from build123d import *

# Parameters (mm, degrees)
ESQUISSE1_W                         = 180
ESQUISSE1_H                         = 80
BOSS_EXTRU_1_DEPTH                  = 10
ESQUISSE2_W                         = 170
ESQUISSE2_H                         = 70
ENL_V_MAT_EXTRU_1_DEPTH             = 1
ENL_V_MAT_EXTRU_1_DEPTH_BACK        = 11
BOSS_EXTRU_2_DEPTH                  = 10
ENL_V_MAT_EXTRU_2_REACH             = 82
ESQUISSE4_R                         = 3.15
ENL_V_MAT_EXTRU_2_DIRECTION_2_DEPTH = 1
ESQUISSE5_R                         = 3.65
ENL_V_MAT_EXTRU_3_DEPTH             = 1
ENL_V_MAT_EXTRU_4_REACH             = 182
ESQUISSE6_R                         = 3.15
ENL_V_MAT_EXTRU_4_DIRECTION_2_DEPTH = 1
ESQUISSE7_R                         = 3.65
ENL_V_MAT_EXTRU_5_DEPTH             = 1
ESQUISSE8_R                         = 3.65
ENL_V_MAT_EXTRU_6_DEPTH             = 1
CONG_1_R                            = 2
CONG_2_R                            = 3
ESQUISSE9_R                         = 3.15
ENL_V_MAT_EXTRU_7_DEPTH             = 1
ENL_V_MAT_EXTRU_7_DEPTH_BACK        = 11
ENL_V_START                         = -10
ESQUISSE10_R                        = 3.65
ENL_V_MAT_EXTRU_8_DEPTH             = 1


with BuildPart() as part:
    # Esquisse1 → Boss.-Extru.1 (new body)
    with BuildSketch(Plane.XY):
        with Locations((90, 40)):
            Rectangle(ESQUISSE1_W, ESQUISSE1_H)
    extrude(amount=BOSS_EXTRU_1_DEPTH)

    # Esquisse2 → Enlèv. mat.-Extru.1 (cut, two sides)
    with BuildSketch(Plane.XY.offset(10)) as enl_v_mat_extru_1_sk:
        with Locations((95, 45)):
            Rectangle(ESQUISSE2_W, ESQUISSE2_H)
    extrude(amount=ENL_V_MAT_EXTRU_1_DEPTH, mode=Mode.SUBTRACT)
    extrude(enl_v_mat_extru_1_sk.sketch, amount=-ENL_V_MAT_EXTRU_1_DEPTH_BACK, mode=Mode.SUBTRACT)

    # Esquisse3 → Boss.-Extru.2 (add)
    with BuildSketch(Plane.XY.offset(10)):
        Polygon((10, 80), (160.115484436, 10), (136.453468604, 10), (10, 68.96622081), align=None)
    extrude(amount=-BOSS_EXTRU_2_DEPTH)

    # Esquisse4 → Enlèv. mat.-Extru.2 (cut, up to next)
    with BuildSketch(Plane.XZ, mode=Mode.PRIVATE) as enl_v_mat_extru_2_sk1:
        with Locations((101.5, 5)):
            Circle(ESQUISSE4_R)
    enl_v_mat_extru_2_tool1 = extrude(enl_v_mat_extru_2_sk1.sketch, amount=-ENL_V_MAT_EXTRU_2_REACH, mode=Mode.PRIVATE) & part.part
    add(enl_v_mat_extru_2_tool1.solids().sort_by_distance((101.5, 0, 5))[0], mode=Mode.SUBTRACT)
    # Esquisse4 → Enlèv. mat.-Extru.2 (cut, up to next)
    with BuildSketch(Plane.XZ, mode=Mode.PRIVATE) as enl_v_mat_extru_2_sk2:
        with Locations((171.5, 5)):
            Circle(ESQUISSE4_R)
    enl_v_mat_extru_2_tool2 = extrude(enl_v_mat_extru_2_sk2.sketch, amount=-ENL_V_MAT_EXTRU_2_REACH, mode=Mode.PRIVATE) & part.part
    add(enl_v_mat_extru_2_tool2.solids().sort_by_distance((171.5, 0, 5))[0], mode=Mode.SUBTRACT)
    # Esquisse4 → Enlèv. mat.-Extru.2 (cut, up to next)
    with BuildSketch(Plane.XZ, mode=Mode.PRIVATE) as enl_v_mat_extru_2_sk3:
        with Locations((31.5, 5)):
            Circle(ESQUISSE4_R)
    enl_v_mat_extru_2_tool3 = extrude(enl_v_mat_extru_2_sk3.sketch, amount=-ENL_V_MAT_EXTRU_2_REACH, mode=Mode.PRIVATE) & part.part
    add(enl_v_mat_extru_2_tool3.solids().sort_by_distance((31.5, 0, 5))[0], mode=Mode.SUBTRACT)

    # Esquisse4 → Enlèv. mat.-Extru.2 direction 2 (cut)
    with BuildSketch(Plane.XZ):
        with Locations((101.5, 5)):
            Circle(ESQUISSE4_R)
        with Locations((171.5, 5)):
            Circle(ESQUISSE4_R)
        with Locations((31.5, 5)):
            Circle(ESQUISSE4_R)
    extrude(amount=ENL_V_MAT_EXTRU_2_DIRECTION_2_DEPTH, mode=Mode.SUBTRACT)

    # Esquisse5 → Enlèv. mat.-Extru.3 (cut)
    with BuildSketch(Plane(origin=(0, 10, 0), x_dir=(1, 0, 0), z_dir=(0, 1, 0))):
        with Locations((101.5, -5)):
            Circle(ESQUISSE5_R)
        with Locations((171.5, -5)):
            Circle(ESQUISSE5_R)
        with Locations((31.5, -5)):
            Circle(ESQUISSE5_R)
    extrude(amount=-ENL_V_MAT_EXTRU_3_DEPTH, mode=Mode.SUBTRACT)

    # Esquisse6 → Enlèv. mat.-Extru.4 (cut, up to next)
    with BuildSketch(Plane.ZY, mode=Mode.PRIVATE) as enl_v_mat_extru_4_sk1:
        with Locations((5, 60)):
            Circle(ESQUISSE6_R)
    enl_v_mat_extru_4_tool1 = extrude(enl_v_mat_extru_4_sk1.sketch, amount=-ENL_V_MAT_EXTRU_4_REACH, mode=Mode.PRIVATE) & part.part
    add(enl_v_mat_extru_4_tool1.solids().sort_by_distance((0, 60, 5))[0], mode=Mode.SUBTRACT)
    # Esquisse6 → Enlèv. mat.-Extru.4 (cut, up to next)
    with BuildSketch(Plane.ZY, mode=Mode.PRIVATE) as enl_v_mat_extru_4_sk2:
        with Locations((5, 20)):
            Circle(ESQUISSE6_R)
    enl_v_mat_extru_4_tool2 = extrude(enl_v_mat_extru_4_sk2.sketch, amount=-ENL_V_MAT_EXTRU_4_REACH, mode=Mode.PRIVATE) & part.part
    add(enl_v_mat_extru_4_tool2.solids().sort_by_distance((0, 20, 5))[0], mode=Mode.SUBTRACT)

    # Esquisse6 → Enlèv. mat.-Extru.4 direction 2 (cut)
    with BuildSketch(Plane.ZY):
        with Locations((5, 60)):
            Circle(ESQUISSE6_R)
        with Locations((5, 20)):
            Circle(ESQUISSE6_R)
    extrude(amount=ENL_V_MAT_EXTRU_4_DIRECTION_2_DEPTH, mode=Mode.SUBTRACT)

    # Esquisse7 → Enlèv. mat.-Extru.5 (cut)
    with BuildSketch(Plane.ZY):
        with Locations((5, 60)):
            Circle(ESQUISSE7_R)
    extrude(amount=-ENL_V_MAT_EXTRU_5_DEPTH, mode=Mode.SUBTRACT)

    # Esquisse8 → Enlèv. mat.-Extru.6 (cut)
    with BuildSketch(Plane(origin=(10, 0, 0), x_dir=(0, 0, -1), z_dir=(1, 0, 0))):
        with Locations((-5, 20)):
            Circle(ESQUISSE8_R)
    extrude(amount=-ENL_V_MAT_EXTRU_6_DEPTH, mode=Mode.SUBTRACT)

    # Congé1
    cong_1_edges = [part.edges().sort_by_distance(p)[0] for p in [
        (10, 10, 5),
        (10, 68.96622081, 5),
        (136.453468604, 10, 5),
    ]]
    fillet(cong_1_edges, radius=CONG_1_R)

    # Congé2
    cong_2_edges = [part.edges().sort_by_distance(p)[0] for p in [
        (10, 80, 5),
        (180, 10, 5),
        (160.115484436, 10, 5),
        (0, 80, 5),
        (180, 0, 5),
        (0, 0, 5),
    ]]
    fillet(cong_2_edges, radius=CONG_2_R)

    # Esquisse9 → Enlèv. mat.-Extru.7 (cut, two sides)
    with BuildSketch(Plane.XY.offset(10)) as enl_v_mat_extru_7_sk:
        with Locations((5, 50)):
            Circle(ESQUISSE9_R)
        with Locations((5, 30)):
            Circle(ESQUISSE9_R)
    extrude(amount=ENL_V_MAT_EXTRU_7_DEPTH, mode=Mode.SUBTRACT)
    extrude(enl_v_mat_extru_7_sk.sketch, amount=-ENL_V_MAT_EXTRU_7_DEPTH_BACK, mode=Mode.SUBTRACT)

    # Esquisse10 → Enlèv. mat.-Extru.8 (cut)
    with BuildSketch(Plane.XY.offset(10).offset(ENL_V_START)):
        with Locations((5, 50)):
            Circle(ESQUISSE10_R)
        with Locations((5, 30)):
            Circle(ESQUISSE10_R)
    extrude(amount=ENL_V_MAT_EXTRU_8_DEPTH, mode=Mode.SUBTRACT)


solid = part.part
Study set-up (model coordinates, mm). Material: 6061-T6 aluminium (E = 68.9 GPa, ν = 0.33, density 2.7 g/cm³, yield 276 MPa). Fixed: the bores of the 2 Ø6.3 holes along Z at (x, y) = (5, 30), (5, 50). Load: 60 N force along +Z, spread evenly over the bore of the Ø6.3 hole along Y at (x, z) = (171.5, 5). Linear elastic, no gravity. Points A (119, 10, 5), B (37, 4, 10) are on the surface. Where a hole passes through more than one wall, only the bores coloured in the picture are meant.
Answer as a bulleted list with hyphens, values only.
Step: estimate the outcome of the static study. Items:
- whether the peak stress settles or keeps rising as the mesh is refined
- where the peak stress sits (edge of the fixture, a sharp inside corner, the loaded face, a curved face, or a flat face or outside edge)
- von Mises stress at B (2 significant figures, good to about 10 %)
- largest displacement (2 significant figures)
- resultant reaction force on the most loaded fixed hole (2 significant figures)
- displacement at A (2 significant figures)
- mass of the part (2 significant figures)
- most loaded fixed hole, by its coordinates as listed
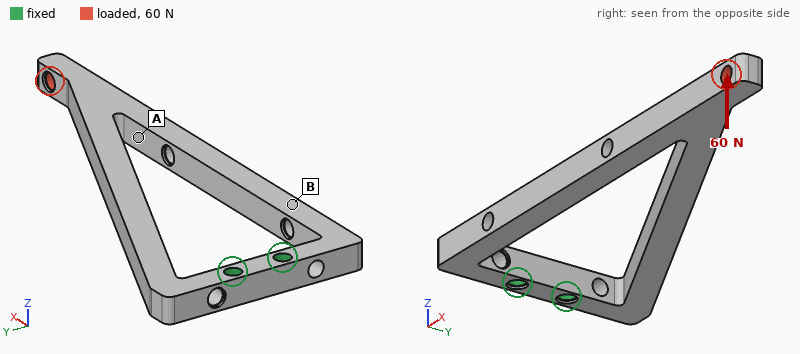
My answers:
- keeps rising
- edge of the fixture
- 27 MPa
- 1.7 mm
- 37 N
- 0.96 mm
- 100 g
- (5, 30)
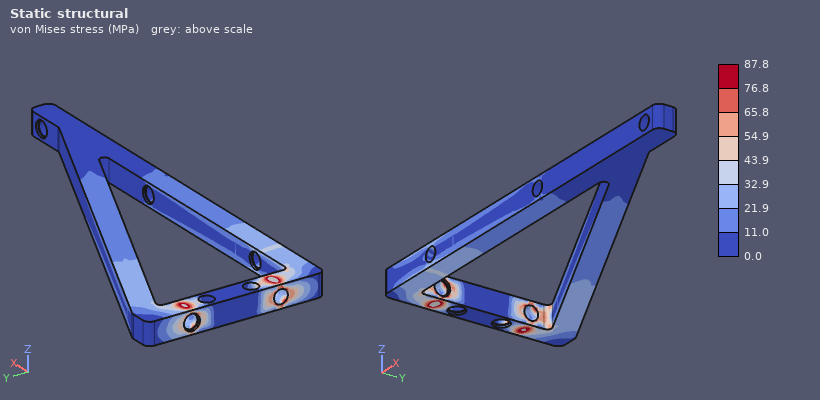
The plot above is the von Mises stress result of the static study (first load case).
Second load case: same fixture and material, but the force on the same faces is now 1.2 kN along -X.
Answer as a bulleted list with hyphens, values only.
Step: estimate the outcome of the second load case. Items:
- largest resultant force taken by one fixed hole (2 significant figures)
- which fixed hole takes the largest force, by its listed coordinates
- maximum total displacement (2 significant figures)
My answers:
- 1.4 kN
- (5, 30)
- 0.54 mm
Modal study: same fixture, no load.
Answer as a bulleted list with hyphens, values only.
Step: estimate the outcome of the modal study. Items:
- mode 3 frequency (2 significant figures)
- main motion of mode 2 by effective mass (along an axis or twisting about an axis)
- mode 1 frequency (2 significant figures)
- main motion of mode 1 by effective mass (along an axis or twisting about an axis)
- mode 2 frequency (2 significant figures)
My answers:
- 1300 Hz
- along Y
- 210 Hz
- along Z
- 560 Hz
